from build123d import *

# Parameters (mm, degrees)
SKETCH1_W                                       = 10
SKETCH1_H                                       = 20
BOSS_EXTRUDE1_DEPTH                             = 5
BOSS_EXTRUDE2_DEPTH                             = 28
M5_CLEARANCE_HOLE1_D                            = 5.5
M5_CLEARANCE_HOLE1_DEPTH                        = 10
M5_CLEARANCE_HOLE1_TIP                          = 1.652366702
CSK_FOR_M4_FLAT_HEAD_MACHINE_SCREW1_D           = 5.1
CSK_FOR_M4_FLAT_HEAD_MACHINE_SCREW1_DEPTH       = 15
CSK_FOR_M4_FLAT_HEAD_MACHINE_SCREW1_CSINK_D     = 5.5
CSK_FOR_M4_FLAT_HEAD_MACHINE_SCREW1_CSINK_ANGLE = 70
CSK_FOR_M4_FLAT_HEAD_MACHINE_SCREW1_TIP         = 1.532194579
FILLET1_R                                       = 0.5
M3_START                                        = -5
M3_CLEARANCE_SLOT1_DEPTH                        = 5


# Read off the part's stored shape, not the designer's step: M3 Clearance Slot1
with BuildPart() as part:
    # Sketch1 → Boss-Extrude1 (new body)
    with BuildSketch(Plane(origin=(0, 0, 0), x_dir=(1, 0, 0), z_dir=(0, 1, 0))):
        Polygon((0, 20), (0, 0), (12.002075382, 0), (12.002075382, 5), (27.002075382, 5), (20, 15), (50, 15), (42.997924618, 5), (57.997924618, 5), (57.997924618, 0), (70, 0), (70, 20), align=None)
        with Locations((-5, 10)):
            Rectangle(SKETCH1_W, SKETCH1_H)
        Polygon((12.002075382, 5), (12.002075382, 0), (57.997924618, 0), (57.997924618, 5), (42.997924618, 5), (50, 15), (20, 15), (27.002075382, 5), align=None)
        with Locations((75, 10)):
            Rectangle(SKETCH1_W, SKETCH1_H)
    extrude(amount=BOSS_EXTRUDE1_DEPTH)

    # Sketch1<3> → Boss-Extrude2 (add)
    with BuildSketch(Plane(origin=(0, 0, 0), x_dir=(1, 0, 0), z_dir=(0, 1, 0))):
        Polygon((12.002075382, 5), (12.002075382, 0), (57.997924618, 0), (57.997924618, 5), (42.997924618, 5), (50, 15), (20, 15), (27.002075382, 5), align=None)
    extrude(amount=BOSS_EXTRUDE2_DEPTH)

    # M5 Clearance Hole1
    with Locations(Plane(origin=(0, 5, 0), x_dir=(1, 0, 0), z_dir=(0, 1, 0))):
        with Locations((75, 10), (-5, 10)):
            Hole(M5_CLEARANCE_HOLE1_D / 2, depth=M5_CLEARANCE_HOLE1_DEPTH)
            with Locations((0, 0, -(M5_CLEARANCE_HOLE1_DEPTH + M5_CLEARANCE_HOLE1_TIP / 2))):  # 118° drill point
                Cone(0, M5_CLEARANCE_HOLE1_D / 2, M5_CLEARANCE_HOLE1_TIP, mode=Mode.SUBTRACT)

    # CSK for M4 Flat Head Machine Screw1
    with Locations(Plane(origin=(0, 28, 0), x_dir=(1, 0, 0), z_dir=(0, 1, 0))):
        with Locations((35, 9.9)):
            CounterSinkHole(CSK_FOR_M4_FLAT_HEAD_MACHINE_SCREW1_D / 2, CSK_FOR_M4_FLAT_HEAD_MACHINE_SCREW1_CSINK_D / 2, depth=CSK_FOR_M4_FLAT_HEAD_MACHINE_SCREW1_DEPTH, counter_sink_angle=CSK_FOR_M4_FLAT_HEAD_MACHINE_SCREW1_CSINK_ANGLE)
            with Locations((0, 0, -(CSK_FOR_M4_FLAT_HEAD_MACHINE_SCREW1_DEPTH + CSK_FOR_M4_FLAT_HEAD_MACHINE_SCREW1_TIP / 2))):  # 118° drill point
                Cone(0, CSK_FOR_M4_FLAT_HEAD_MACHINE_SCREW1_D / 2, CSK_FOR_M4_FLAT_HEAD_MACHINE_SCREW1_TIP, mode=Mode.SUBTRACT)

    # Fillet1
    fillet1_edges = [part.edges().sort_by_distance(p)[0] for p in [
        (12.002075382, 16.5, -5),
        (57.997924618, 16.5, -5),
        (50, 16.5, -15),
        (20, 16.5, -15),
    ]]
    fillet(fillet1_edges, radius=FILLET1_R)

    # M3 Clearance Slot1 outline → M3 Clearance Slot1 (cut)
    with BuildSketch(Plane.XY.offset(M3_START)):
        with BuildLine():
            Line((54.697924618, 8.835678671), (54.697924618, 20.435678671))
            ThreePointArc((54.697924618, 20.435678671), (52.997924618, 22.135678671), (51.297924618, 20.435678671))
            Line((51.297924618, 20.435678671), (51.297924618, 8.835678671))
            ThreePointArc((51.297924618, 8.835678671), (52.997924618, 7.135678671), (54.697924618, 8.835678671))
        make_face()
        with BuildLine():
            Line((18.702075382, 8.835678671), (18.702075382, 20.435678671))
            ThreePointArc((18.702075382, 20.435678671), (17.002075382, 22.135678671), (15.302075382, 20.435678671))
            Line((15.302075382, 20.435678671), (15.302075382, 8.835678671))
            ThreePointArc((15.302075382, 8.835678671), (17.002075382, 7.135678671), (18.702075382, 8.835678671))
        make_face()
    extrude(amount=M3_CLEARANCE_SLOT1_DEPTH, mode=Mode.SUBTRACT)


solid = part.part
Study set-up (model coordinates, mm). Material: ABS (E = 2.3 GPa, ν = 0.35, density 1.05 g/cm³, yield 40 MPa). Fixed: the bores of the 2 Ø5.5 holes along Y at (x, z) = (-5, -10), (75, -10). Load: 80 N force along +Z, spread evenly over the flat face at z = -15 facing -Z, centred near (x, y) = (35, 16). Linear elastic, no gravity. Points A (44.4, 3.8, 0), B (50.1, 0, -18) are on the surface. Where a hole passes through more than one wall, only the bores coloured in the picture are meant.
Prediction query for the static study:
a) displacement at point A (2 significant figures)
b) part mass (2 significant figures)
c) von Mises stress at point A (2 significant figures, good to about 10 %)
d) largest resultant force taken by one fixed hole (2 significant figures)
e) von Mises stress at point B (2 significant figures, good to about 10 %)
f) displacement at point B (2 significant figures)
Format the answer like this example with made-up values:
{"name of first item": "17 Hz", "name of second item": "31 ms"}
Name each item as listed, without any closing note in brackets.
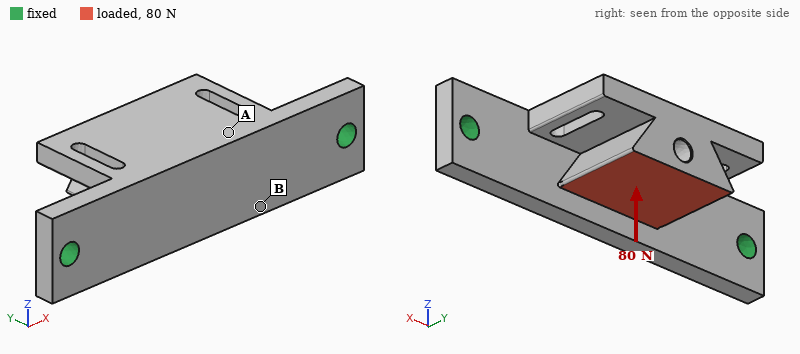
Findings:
{"displacement at point A": "0.18 mm", "part mass": "19 g", "von Mises stress at point A": "1.8 MPa", "largest resultant force taken by one fixed hole": "40 N", "von Mises stress at point B": "4.2 MPa", "displacement at point B": "0.17 mm"}
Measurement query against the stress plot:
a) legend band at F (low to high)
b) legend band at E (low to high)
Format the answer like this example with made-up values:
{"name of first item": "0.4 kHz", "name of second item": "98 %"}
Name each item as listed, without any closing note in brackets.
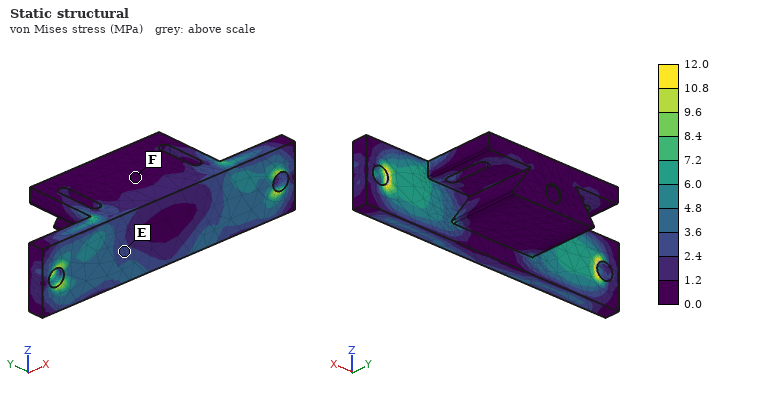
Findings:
{"legend band at F": "0.0 to 1.2 MPa", "legend band at E": "2.4 to 3.6 MPa"}
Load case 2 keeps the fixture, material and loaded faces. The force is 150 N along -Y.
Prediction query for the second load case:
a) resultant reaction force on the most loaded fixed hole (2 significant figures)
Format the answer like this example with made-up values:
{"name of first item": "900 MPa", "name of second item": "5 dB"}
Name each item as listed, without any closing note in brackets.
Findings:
{"resultant reaction force on the most loaded fixed hole": "84 N"}
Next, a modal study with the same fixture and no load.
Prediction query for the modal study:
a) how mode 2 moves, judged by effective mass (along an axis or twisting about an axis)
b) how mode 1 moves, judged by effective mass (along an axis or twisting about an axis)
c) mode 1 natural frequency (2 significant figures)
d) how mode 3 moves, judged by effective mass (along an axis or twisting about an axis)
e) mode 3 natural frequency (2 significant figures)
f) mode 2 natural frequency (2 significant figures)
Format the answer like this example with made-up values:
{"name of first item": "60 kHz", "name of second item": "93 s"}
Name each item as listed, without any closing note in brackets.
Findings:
{"how mode 2 moves, judged by effective mass": "along Y", "how mode 1 moves, judged by effective mass": "along Z", "mode 1 natural frequency": "670 Hz", "how mode 3 moves, judged by effective mass": "along X", "mode 3 natural frequency": "1800 Hz", "mode 2 natural frequency": "1100 Hz"}
